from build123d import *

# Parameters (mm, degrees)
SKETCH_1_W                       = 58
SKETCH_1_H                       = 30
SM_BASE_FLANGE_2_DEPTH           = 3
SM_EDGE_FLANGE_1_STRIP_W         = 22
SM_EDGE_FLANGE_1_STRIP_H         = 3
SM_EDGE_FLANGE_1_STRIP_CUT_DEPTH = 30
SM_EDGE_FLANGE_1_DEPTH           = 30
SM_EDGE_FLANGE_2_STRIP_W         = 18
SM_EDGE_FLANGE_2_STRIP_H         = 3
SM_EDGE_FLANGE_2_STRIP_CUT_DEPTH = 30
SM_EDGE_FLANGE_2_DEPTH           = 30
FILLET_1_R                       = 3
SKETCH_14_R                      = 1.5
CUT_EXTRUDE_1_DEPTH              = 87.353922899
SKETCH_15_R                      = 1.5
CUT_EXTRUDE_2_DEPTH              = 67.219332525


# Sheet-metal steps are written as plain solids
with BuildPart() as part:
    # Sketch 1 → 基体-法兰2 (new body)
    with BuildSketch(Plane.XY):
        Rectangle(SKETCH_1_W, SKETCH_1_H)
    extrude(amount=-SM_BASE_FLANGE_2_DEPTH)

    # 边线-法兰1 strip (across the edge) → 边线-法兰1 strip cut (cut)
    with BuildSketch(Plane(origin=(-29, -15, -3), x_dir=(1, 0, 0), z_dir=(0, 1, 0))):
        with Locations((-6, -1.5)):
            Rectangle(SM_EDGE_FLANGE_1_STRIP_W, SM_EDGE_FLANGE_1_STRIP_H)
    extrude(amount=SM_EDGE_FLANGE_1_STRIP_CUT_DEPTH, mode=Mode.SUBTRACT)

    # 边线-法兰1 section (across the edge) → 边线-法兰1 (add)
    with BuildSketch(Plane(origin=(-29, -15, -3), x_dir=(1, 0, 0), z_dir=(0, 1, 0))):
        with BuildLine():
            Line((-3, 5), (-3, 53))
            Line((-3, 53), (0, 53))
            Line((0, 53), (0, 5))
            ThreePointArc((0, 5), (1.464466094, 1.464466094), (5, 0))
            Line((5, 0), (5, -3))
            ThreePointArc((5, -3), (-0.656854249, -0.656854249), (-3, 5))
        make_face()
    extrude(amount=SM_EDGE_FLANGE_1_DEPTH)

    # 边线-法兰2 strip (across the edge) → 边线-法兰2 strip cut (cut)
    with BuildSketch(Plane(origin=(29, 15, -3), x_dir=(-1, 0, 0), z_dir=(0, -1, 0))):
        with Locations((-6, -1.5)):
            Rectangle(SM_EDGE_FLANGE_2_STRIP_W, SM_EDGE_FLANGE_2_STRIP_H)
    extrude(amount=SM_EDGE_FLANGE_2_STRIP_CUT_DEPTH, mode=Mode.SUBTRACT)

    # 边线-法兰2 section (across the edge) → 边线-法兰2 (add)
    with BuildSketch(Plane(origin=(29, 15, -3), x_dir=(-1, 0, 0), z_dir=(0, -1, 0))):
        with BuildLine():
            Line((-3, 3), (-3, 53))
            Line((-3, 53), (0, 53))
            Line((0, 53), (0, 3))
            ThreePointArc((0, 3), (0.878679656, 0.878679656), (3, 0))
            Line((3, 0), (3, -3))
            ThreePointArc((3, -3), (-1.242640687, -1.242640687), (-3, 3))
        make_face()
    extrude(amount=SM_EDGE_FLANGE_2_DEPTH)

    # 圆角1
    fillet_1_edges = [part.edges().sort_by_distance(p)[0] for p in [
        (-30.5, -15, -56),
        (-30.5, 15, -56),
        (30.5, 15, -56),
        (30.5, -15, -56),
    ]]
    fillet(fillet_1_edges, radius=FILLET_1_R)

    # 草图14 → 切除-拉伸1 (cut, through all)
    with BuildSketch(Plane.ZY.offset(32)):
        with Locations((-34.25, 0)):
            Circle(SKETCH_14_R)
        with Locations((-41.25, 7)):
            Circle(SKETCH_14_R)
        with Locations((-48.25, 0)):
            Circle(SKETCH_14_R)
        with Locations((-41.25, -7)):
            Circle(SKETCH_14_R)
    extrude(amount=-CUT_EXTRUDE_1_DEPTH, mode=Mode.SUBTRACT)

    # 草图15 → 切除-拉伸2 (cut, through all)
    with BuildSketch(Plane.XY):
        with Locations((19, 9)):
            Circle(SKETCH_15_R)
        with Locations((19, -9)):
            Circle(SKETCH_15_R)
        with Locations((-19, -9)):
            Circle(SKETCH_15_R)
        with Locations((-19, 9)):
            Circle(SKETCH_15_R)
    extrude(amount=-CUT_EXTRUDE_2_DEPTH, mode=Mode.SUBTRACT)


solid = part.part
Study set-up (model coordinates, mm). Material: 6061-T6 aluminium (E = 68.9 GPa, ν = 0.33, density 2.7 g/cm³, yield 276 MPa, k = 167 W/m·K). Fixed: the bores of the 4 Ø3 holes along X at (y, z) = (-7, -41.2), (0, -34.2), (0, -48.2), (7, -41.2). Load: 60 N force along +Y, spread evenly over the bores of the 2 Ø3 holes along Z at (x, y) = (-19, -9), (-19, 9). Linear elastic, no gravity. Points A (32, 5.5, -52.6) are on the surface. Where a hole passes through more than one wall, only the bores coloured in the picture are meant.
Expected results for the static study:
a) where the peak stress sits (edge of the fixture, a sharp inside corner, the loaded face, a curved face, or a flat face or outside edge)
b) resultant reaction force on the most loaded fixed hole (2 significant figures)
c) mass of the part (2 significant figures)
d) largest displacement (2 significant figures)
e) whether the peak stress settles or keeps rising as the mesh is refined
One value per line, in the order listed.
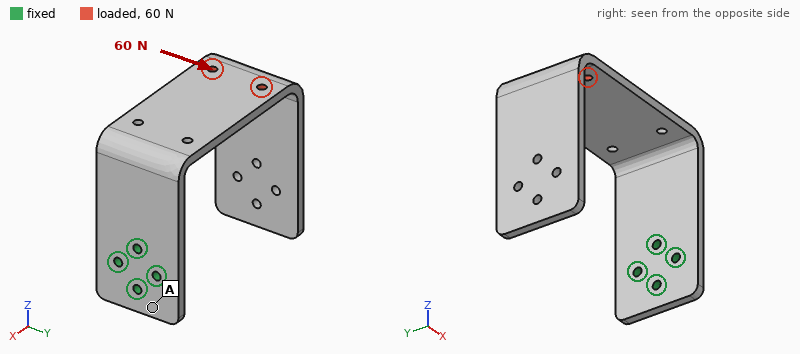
edge of the fixture
120 N
39 g
0.93 mm
keeps rising
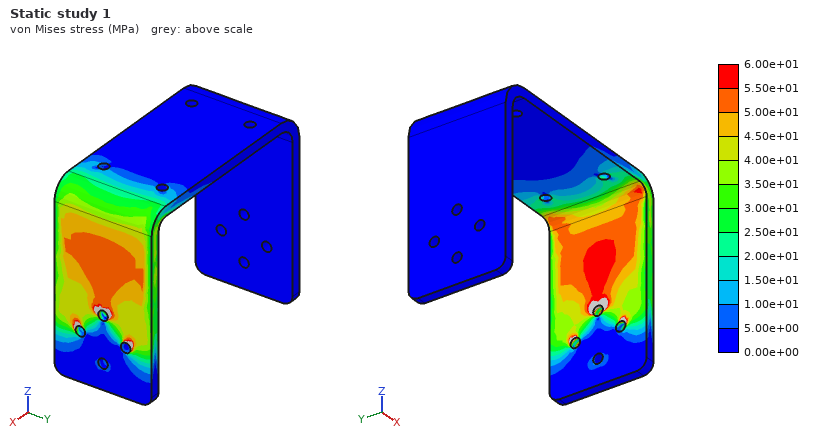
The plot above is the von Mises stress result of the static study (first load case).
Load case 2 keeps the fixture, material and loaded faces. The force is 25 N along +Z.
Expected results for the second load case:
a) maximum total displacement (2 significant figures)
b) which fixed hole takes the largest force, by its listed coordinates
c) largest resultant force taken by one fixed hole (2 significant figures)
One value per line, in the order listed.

1.0 mm
(0, -34.2)
95 N
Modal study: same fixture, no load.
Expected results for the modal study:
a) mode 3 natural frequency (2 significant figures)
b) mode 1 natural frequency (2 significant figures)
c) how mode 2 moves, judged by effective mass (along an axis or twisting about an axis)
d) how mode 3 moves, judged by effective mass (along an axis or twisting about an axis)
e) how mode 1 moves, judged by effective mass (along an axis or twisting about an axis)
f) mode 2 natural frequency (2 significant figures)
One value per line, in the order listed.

480 Hz
180 Hz
along Y
along X
along Z
260 Hz
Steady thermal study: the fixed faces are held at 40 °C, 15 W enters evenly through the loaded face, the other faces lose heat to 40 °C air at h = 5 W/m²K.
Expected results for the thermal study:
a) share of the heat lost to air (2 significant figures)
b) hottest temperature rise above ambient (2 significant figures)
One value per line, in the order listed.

17 %
74 K
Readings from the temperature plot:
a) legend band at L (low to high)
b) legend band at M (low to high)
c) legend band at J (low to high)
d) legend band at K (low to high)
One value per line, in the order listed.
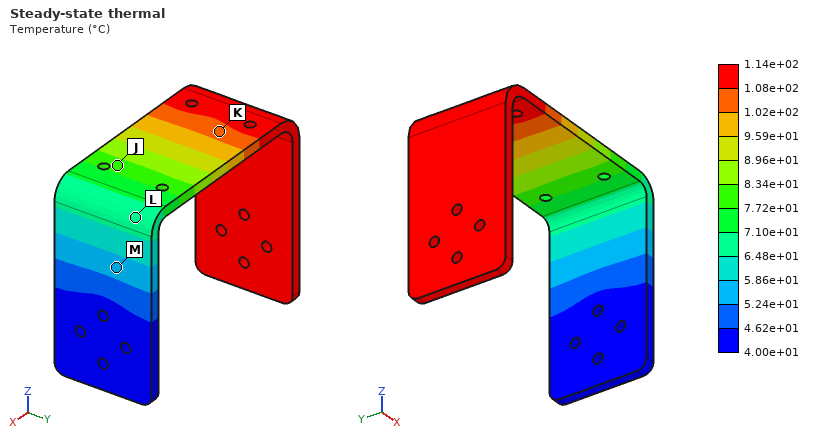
6.48e+01 to 7.10e+01 °C
5.24e+01 to 5.86e+01 °C
7.72e+01 to 8.34e+01 °C
1.02e+02 to 1.08e+02 °C
